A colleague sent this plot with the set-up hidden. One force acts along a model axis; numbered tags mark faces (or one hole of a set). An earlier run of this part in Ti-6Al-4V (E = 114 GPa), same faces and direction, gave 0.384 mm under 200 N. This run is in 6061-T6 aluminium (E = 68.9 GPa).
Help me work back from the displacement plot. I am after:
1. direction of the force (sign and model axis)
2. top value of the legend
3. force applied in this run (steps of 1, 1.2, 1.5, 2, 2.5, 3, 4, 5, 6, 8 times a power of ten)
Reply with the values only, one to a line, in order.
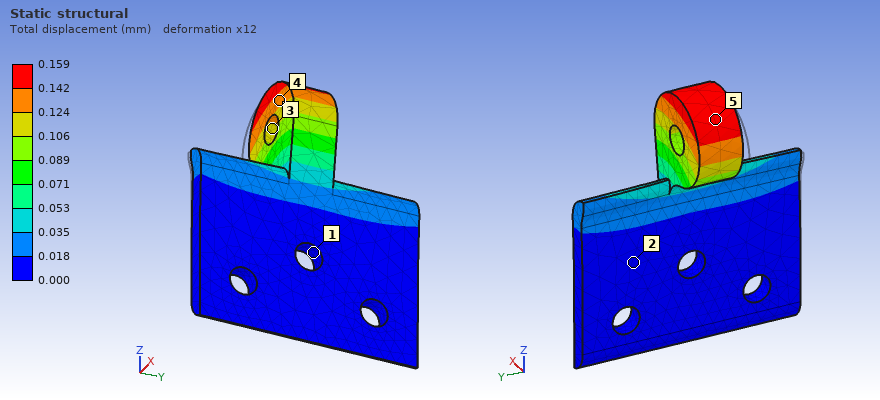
+X
0.159 mm
50 N
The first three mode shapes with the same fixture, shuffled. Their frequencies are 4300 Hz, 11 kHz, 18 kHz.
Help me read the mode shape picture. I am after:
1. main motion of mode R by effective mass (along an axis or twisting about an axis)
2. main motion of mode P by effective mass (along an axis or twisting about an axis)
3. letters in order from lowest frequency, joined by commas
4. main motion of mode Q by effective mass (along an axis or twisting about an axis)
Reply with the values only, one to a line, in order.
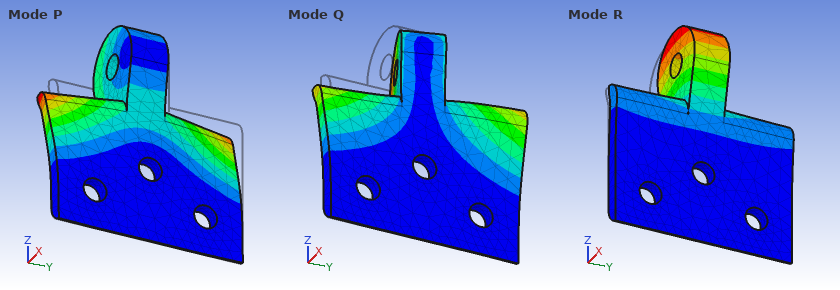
along X
along X
R, Q, P
along Y
